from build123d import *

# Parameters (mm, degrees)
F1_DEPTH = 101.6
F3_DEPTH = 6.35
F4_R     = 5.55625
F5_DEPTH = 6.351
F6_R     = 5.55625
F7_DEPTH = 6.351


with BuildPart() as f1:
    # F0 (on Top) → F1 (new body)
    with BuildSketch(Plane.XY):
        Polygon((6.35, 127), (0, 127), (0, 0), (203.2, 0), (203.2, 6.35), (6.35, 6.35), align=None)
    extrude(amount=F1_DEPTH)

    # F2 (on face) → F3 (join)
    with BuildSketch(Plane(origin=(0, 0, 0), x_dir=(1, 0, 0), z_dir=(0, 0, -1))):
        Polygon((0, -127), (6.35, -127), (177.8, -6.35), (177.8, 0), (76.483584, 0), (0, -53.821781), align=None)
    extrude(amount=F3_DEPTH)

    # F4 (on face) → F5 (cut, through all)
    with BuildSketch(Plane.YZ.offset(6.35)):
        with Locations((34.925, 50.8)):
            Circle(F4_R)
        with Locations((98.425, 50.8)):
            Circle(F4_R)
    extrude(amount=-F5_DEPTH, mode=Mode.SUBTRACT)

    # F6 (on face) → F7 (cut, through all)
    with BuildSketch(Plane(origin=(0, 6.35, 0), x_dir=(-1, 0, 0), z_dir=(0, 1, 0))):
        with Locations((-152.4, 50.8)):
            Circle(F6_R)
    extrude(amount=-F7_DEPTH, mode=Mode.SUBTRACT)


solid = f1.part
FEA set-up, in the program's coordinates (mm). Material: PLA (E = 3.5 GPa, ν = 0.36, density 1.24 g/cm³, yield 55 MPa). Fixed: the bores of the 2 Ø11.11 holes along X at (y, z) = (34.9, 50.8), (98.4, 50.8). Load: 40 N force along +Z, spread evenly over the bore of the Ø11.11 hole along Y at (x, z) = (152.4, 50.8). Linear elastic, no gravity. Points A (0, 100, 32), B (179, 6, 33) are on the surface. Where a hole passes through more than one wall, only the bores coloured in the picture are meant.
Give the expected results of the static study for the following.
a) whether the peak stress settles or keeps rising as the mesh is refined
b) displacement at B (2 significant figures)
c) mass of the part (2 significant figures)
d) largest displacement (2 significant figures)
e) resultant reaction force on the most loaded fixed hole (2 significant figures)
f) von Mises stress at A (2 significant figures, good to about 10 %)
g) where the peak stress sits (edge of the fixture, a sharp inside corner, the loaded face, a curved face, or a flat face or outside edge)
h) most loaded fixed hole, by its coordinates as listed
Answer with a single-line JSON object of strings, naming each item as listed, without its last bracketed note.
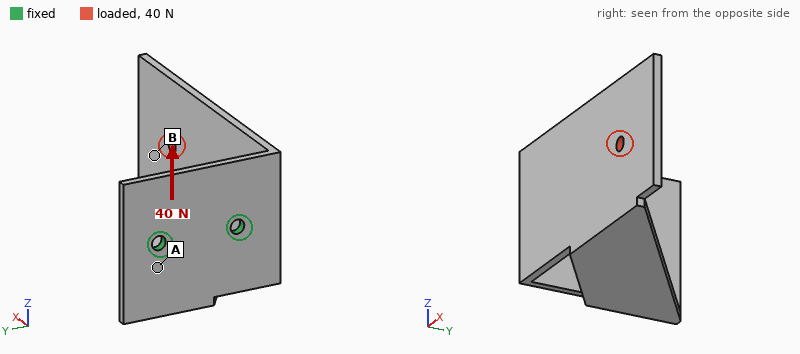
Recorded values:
{"whether the peak stress settles or keeps rising as the mesh is refined": "keeps rising", "displacement at B": "2.2 mm", "mass of the part": "340 g", "largest displacement": "2.5 mm", "resultant reaction force on the most loaded fixed hole": "56 N", "von Mises stress at A": "2.1 MPa", "where the peak stress sits": "edge of the fixture", "most loaded fixed hole, by its coordinates as listed": "(34.9, 50.8)"}
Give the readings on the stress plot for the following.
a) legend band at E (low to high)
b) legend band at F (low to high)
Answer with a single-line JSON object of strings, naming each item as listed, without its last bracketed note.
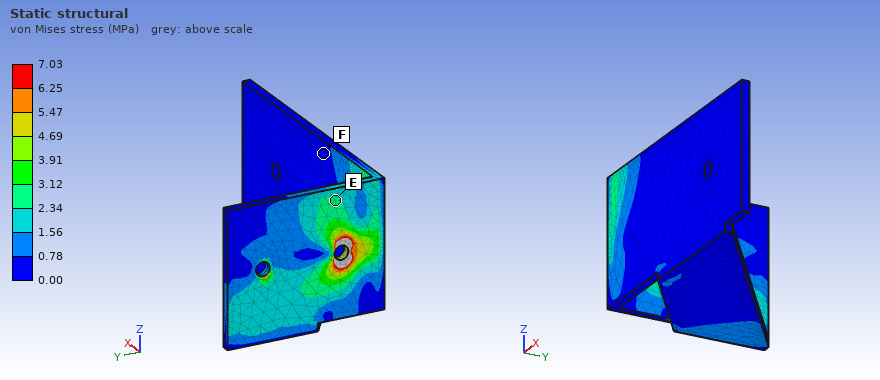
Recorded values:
{"legend band at E": "2.34 to 3.12 MPa", "legend band at F": "0.00 to 0.78 MPa"}
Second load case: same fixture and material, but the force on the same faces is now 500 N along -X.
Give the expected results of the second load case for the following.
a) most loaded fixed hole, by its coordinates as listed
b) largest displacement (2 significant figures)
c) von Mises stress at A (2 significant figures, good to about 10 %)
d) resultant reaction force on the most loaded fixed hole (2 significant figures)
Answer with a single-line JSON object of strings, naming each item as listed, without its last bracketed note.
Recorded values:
{"most loaded fixed hole, by its coordinates as listed": "(34.9, 50.8)", "largest displacement": "2.9 mm", "von Mises stress at A": "3.5 MPa", "resultant reaction force on the most loaded fixed hole": "600 N"}
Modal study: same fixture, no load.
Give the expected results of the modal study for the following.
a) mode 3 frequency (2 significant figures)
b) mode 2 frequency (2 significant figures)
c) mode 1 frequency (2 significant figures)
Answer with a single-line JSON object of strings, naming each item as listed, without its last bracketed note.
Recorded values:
{"mode 3 frequency": "220 Hz", "mode 2 frequency": "80 Hz", "mode 1 frequency": "62 Hz"}
